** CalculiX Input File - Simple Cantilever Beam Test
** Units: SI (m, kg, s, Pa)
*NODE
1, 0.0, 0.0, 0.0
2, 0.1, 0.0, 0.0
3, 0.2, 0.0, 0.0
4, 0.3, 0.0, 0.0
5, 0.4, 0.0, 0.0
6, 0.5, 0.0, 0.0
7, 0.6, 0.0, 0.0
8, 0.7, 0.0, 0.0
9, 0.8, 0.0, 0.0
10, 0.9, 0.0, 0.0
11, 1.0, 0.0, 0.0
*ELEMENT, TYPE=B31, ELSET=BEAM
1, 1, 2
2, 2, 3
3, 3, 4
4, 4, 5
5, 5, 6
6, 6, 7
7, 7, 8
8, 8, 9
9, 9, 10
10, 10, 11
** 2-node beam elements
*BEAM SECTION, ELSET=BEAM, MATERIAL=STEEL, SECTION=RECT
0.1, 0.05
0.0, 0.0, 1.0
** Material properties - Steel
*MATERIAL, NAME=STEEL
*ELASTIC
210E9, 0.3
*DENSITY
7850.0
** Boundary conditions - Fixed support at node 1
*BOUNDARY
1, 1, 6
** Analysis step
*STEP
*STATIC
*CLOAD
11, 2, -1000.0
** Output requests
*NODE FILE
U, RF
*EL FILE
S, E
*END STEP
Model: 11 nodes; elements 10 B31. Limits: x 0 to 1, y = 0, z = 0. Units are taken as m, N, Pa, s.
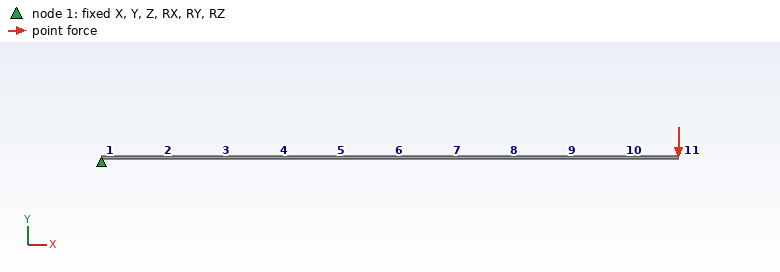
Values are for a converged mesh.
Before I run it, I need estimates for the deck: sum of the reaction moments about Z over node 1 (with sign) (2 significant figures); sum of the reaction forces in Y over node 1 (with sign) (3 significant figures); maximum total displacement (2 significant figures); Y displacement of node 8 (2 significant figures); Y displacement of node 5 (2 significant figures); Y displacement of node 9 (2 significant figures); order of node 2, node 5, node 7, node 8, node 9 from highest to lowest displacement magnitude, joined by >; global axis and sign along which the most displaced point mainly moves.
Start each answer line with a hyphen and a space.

- 1000 N·m
- 1000 N
- 0.0015 m
- -8.6e-04 m
- -3.2e-04 m
- -0.0011 m
- node 9 > node 8 > node 7 > node 5 > node 2
- -Y
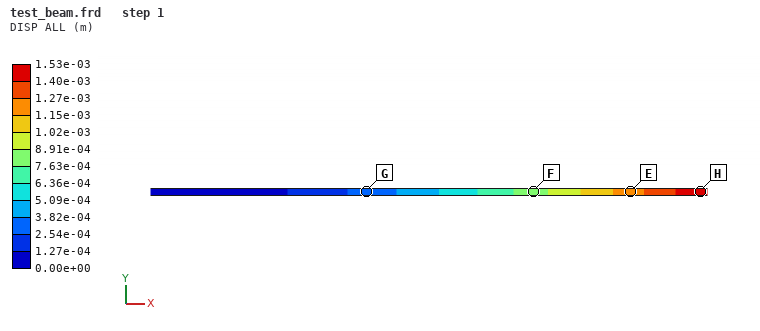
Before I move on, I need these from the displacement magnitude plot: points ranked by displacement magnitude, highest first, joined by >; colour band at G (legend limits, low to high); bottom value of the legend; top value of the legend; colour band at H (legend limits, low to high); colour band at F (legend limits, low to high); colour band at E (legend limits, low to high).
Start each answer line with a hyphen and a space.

- H > E > F > G
- 2.54e-04 to 3.82e-04 m
- 0.00e+00 m
- 1.53e-03 m
- 1.40e-03 to 1.53e-03 m
- 7.63e-04 to 8.91e-04 m
- 1.15e-03 to 1.27e-03 m
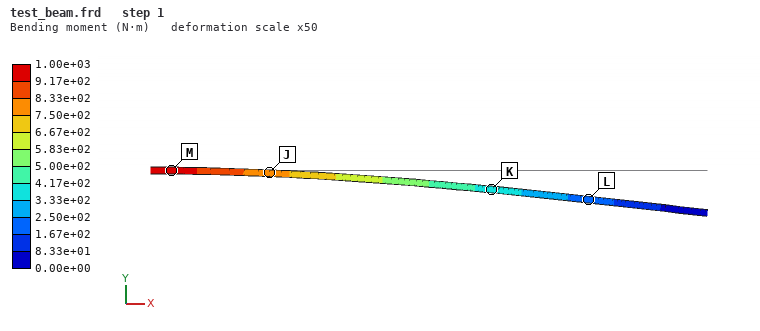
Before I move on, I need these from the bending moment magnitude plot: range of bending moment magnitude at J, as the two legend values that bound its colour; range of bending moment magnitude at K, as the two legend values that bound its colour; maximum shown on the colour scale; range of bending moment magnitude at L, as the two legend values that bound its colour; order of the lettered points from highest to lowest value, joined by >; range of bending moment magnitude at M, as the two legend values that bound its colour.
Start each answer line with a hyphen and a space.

- 7.50e+02 to 8.33e+02 N·m
- 3.33e+02 to 4.17e+02 N·m
- 1.00e+03 N·m
- 1.67e+02 to 2.50e+02 N·m
- M > J > K > L
- 9.17e+02 to 1.00e+03 N·m
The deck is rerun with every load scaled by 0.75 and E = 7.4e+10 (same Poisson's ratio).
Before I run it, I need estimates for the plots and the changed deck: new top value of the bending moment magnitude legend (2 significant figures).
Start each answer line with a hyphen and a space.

- 750 N·m
